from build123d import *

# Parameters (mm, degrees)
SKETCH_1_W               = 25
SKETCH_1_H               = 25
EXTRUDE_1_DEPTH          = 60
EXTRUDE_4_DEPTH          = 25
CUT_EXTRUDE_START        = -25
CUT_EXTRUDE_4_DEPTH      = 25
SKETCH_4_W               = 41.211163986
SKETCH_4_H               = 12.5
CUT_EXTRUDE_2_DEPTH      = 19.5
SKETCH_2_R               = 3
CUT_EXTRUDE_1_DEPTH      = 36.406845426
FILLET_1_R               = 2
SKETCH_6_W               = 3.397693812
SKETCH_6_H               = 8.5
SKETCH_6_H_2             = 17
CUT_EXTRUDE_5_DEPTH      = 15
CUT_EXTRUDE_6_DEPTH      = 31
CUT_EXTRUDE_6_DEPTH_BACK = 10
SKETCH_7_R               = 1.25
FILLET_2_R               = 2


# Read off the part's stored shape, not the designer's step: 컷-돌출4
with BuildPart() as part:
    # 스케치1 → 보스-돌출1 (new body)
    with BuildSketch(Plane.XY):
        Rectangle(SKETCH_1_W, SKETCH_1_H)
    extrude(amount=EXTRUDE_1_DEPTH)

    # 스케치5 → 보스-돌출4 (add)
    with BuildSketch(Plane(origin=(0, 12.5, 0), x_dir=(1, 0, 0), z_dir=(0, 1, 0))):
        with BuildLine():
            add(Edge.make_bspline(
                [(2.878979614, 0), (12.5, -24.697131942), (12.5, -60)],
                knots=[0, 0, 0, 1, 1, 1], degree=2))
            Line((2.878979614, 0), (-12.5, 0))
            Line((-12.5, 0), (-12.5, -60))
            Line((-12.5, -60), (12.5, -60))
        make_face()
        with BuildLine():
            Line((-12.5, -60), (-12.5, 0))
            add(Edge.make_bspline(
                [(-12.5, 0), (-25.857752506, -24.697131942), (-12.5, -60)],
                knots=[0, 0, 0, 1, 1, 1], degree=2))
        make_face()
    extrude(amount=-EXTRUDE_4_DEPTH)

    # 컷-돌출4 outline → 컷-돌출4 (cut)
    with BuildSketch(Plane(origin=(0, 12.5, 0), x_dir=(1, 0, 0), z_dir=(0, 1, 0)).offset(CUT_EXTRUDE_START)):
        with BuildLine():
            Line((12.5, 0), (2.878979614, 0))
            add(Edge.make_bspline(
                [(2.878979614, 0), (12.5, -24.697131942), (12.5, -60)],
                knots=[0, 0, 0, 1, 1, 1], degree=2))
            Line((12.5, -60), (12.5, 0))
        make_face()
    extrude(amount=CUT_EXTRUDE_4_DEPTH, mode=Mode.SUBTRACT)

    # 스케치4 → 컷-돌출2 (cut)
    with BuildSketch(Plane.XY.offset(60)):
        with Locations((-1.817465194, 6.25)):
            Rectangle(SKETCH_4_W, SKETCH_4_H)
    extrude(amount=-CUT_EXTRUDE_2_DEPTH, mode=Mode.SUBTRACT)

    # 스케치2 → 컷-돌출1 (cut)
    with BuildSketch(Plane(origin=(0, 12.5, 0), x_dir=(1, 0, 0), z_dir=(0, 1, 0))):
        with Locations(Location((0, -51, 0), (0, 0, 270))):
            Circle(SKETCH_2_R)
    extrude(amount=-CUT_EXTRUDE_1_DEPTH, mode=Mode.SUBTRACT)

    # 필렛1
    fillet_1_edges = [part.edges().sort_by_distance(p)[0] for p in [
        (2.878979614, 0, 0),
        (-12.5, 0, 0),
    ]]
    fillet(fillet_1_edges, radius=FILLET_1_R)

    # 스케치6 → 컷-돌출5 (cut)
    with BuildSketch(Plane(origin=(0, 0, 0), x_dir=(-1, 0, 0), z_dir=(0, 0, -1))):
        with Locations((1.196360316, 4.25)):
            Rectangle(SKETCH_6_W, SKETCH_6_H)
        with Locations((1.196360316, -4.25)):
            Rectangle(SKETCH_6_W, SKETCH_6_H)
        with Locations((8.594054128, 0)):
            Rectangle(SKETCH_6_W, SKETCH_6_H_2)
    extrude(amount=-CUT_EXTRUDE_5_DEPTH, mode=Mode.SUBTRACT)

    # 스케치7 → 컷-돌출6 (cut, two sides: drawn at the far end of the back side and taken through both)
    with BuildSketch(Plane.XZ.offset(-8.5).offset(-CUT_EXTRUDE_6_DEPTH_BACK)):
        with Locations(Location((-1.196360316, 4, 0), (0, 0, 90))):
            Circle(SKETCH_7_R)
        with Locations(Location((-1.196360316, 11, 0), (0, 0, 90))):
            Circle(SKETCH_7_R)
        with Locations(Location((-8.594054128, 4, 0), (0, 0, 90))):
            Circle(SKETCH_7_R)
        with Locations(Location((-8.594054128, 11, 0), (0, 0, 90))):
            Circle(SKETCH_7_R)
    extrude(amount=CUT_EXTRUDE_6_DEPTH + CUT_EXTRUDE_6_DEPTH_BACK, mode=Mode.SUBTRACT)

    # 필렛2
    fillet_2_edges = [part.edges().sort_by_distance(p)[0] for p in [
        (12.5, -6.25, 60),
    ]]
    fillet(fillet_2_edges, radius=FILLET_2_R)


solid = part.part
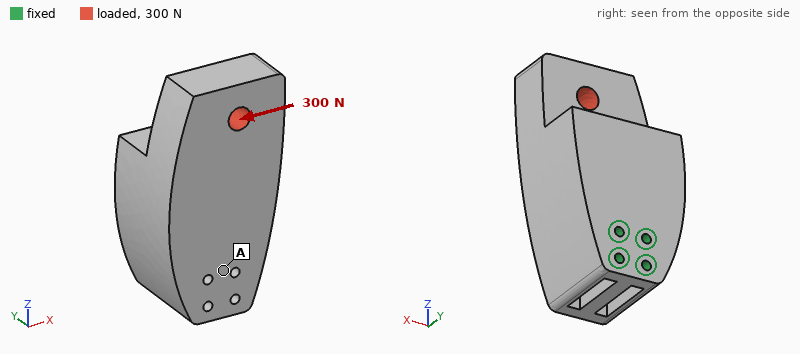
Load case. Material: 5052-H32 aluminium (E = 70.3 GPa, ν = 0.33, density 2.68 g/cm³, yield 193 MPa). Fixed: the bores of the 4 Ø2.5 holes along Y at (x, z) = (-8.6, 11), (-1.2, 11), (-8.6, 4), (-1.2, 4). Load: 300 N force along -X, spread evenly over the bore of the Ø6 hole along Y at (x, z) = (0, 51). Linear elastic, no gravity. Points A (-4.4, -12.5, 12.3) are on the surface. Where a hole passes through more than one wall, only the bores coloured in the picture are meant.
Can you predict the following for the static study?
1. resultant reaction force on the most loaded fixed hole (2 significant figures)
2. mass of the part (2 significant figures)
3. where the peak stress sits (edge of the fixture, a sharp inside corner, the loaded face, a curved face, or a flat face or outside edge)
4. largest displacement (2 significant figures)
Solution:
740 N
82 g
edge of the fixture
27 µm
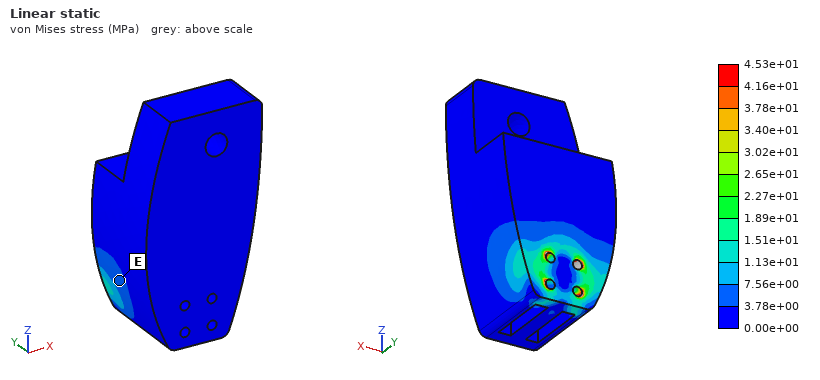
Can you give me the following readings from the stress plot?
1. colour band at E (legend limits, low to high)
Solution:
3.78e+00 to 7.56e+00 MPa
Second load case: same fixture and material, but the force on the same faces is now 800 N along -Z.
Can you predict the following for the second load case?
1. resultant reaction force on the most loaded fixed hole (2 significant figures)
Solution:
740 N
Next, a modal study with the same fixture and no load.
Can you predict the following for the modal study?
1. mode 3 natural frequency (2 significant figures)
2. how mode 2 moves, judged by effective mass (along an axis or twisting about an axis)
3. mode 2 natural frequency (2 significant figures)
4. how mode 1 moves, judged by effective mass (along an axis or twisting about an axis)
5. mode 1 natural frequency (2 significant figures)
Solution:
5900 Hz
along X
3400 Hz
along Y
2600 Hz
